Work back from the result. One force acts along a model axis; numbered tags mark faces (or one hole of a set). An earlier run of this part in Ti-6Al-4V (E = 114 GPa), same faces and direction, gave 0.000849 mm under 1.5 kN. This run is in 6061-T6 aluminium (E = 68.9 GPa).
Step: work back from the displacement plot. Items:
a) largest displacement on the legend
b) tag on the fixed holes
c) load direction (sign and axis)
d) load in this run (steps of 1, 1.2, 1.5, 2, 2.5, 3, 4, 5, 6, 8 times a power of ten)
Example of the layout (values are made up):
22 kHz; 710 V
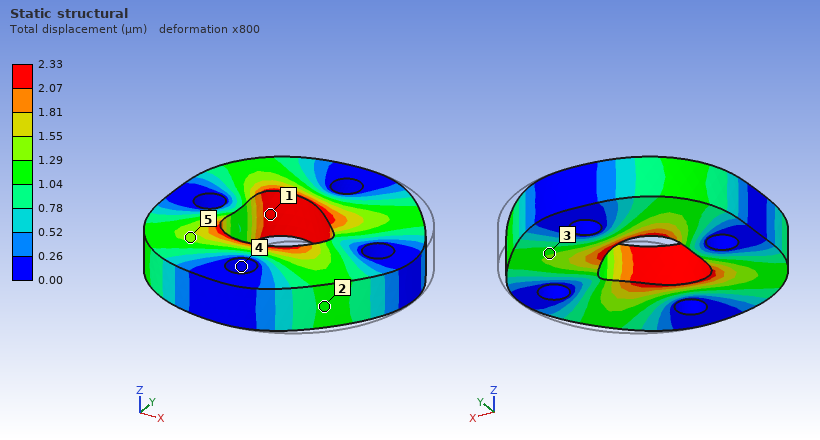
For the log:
2.33 µm; 4; -X; 2.5 kN
